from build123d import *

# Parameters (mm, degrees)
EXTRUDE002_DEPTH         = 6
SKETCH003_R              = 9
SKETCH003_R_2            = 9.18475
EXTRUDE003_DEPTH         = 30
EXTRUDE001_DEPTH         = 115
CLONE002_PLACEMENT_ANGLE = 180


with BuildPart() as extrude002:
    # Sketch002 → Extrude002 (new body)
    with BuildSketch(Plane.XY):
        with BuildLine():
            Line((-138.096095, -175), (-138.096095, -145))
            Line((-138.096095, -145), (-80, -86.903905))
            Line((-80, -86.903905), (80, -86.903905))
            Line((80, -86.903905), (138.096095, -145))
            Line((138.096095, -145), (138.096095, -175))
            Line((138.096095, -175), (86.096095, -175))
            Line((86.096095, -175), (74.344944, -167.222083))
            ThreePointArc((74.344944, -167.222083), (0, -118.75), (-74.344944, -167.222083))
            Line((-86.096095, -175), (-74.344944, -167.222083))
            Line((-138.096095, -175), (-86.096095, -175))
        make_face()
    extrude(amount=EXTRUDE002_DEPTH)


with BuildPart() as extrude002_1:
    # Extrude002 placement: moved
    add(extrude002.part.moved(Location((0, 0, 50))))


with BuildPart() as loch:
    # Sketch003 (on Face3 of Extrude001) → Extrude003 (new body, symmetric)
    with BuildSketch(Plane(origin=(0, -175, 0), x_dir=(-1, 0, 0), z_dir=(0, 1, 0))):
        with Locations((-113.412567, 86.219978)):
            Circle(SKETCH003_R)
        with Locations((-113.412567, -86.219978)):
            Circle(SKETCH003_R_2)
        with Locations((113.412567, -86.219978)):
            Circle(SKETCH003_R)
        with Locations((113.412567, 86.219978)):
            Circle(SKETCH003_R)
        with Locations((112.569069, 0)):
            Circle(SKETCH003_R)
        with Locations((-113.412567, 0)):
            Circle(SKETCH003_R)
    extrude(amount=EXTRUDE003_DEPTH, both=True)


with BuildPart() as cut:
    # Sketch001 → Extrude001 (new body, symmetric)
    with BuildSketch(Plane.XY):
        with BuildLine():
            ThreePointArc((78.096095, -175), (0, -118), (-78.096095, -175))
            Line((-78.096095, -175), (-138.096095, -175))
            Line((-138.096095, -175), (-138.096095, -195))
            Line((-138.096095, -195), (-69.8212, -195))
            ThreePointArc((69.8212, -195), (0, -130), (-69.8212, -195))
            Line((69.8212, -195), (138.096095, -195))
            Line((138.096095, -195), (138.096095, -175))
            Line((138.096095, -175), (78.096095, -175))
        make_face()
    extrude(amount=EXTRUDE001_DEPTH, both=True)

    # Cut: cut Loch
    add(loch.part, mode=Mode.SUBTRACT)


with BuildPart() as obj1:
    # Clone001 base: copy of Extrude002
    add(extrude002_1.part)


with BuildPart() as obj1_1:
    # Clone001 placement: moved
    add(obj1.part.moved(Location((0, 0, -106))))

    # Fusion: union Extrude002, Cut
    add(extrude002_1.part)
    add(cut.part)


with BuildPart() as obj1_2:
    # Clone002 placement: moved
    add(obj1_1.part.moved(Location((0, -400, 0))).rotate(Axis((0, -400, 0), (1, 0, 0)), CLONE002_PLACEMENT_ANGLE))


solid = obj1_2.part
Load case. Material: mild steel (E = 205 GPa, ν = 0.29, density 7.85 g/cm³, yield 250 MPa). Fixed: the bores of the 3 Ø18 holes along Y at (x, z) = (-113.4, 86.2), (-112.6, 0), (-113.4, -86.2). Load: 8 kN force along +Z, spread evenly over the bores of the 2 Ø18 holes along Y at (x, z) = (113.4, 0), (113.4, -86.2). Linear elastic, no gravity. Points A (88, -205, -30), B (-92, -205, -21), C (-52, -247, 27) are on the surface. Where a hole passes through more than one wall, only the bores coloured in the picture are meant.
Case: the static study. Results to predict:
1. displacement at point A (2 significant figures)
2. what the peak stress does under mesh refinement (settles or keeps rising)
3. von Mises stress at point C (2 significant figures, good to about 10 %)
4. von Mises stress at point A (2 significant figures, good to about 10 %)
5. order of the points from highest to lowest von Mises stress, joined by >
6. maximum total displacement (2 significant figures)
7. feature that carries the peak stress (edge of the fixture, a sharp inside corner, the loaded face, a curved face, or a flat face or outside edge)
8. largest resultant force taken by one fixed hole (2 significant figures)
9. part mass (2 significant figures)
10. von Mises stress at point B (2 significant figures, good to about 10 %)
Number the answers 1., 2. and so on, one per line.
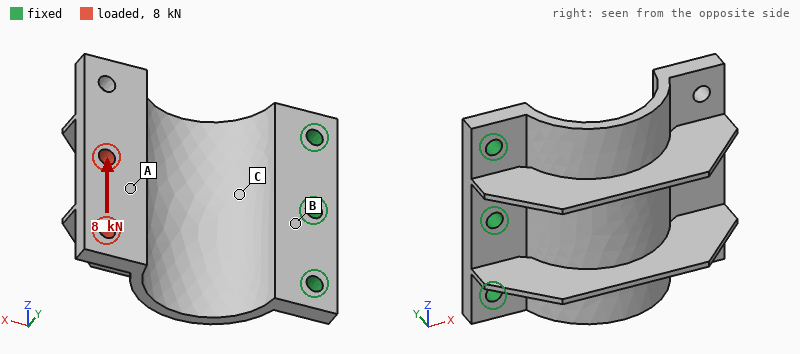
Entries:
1. 0.31 mm
2. keeps rising
3. 48 MPa
4. 13 MPa
5. C > B > A
6. 0.47 mm
7. edge of the fixture
8. 11 kN
9. 10 kg
10. 29 MPa
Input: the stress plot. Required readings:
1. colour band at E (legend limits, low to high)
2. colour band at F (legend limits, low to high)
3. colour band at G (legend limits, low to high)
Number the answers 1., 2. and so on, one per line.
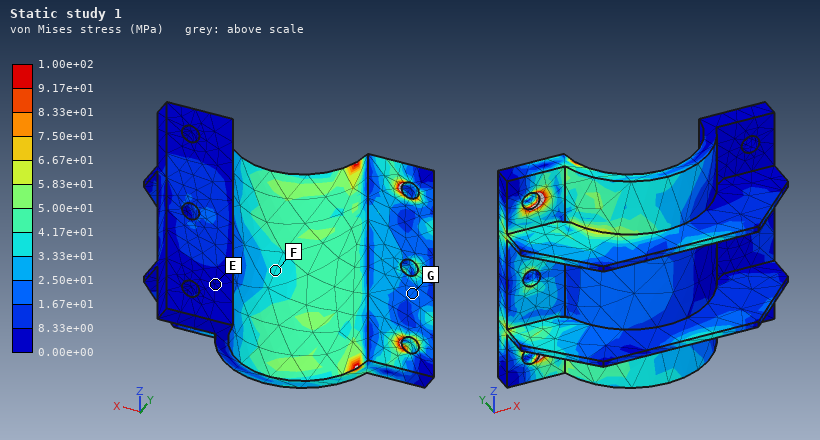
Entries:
1. 0.00e+00 to 8.33e+00 MPa
2. 3.33e+01 to 4.17e+01 MPa
3. 1.67e+01 to 2.50e+01 MPa
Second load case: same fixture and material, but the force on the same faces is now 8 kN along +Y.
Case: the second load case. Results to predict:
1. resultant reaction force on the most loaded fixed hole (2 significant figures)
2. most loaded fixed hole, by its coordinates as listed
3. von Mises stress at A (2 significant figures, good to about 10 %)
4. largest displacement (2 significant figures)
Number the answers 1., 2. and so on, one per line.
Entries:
1. 5.3 kN
2. (-112.6, 0)
3. 22 MPa
4. 1.0 mm
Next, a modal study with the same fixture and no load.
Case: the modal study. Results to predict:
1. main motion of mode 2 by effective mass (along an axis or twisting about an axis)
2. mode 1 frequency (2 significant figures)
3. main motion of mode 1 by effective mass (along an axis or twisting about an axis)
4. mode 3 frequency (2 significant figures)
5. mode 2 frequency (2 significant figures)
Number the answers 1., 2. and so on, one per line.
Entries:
1. along Z
2. 300 Hz
3. along Y
4. 730 Hz
5. 360 Hz
